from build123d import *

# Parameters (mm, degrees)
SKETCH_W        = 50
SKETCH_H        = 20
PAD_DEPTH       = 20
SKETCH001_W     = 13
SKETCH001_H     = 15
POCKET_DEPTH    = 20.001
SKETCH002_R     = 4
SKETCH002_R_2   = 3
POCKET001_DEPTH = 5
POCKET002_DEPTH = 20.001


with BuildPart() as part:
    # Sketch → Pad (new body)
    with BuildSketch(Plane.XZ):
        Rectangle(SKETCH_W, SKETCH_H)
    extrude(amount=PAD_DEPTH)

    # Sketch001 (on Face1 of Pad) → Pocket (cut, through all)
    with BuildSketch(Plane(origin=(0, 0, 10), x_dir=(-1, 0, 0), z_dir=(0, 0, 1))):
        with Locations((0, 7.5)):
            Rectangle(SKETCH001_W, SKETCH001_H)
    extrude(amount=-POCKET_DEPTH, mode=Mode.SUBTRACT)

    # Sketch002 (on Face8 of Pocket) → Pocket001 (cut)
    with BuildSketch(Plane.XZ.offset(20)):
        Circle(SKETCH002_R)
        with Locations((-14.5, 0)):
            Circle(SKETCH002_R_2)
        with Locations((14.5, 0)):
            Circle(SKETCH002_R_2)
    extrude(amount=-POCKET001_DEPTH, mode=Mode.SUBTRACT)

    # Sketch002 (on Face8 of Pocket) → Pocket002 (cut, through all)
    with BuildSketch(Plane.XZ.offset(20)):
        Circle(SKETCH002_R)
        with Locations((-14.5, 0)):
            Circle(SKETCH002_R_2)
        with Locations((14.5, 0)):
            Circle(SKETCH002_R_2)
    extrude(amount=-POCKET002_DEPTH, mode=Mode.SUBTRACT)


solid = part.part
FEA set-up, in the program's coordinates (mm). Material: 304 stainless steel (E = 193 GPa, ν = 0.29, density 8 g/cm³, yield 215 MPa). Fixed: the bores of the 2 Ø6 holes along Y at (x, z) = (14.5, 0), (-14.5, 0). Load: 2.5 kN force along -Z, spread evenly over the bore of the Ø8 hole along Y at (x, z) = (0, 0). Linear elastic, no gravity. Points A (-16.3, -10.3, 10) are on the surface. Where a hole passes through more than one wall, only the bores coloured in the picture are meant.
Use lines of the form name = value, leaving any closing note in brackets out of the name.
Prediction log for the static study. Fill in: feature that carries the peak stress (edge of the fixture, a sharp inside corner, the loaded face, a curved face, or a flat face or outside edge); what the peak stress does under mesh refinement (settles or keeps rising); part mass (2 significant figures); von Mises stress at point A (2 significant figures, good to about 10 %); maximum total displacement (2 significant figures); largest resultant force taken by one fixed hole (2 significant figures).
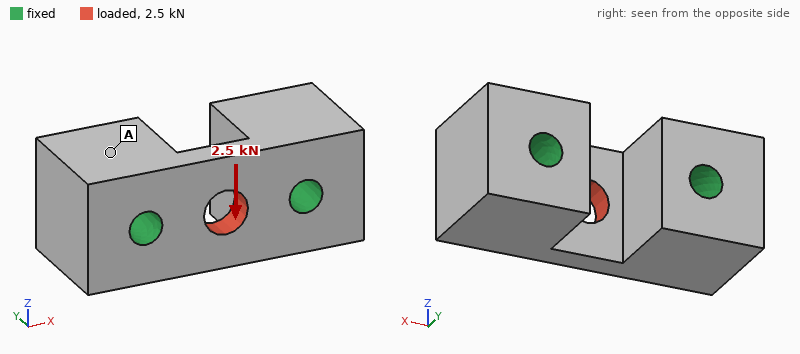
feature that carries the peak stress = edge of the fixture
what the peak stress does under mesh refinement = keeps rising
part mass = 120 g
von Mises stress at point A = 4.1 MPa
maximum total displacement = 2.6 µm
largest resultant force taken by one fixed hole = 1.3 kN
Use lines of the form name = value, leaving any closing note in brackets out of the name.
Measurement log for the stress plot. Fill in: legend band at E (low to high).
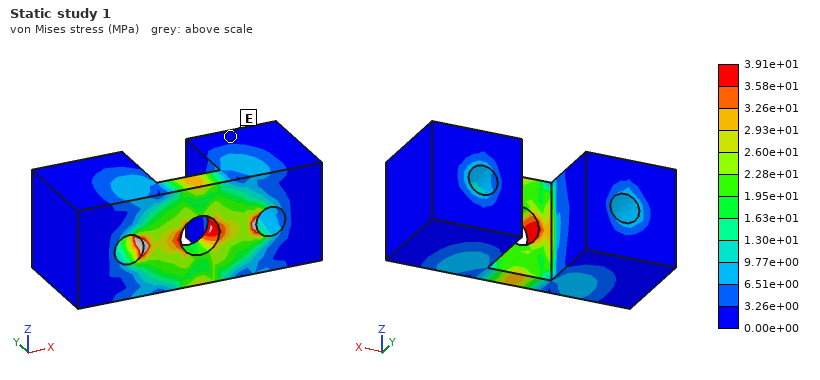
legend band at E = 0.00e+00 to 3.26e+00 MPa
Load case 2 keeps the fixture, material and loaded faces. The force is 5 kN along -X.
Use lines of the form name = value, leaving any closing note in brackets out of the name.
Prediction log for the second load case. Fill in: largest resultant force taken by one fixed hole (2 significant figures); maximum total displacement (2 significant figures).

largest resultant force taken by one fixed hole = 2.5 kN
maximum total displacement = 2.2 µm
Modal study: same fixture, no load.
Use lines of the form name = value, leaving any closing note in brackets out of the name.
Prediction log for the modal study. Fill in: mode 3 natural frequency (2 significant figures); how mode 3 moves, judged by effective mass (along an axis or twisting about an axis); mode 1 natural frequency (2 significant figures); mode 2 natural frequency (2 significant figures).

mode 3 natural frequency = 53 kHz
how mode 3 moves, judged by effective mass = along Y
mode 1 natural frequency = 39 kHz
mode 2 natural frequency = 39 kHz
